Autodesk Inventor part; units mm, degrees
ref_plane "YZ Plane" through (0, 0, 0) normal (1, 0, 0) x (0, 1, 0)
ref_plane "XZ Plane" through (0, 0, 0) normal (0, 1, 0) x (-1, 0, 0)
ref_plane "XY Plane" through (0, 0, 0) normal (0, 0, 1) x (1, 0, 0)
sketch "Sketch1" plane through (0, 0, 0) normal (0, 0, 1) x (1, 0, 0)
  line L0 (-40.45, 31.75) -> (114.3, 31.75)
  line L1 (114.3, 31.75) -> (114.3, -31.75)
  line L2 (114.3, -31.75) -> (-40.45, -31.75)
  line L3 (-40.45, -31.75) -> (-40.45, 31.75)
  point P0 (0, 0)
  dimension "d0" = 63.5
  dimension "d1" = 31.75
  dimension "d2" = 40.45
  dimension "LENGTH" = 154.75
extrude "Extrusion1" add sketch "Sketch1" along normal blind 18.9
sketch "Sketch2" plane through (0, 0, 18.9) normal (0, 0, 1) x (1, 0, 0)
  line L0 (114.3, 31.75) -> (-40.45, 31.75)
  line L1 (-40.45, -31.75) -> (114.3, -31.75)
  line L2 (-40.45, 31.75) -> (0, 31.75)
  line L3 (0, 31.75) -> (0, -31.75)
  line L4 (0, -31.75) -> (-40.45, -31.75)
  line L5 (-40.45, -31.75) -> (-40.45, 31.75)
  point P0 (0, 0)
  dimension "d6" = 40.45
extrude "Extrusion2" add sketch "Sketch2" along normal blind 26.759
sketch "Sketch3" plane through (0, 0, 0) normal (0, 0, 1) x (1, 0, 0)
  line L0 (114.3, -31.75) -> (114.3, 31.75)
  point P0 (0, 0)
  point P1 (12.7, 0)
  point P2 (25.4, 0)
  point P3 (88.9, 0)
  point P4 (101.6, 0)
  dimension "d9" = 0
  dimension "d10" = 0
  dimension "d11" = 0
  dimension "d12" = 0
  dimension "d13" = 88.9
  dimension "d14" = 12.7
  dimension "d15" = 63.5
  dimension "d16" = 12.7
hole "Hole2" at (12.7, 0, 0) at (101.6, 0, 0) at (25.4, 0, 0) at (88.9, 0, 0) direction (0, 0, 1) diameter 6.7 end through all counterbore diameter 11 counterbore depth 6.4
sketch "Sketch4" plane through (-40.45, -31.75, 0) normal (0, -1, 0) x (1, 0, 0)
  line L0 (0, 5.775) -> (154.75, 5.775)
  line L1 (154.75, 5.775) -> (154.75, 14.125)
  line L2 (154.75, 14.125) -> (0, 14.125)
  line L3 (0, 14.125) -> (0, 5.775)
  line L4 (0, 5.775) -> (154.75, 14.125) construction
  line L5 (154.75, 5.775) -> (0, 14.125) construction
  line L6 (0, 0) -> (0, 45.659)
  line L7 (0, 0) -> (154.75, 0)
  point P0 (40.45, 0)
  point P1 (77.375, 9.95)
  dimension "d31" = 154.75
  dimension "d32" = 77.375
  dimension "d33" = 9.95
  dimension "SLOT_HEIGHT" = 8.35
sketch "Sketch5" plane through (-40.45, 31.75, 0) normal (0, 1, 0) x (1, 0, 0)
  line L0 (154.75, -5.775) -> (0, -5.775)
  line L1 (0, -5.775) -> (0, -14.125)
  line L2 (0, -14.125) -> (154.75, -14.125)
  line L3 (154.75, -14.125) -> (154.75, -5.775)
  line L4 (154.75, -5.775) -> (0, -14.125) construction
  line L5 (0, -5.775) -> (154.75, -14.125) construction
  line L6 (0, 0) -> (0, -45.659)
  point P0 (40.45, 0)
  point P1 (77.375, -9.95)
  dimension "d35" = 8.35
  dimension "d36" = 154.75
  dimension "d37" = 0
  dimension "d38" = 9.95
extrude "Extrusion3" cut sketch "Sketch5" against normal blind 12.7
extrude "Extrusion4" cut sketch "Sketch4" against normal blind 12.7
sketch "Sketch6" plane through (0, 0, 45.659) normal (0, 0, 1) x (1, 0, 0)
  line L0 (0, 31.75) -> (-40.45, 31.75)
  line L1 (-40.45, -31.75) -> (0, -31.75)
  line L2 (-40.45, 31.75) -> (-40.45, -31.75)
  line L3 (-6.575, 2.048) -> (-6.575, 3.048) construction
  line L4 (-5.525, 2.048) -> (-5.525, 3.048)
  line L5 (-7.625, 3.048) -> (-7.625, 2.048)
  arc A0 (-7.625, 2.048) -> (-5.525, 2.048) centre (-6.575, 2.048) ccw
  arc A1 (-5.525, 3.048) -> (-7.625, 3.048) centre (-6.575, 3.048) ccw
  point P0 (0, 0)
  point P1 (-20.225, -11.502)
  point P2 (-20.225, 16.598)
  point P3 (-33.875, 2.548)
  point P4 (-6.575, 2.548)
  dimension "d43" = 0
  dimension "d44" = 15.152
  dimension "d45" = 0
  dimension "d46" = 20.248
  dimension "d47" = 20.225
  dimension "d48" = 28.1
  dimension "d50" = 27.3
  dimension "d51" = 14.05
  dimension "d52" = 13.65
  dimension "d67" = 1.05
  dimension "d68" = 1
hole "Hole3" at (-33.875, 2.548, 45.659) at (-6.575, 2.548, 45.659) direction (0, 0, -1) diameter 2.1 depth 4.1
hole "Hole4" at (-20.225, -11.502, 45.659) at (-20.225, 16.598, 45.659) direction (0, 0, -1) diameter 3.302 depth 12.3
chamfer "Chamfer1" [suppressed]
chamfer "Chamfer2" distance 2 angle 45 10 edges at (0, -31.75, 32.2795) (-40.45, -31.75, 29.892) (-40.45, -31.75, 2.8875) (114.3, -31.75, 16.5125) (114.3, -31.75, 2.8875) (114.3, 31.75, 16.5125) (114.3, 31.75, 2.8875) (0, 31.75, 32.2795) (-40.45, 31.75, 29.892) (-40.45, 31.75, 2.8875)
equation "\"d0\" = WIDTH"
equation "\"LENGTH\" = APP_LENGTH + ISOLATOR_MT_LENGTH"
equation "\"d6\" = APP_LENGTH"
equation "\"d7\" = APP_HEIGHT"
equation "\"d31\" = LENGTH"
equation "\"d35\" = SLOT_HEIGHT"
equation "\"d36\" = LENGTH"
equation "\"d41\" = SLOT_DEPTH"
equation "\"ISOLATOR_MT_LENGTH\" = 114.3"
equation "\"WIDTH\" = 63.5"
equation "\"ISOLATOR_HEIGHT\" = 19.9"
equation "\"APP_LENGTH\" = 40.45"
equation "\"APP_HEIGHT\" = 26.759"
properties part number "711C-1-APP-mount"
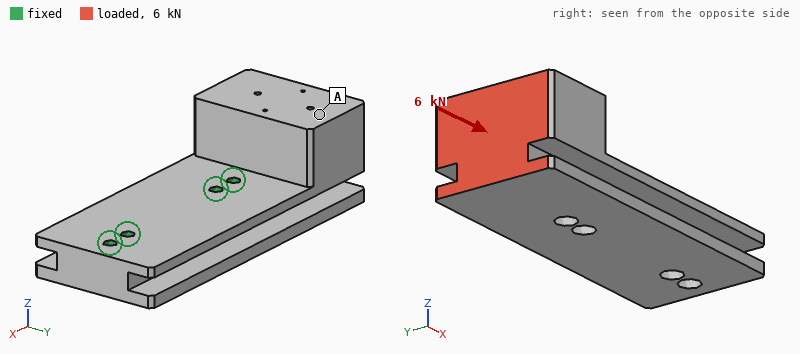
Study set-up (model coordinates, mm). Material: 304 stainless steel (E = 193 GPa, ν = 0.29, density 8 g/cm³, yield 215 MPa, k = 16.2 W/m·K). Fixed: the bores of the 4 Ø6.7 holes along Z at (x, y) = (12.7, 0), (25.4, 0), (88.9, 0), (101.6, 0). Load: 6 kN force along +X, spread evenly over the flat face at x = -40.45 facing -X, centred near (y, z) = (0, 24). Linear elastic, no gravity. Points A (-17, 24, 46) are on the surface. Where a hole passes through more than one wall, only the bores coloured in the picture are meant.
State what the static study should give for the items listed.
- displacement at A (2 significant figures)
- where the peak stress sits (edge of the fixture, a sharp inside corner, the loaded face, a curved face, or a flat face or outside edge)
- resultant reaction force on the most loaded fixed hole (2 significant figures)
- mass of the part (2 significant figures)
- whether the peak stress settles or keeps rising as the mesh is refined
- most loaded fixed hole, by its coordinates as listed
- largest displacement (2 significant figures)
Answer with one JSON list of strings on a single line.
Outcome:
["20 µm", "edge of the fixture", "4.9 kN", "1.7 kg", "keeps rising", "(12.7, 0)", "27 µm"]
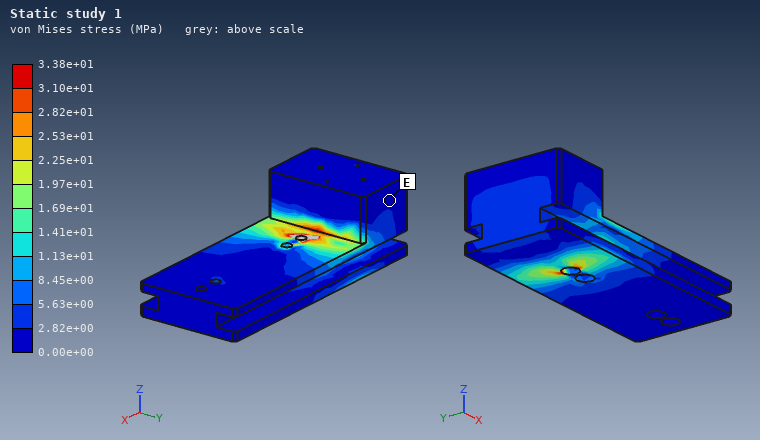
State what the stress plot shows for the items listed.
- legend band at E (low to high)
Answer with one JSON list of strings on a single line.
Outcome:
["0.00e+00 to 2.82e+00 MPa"]
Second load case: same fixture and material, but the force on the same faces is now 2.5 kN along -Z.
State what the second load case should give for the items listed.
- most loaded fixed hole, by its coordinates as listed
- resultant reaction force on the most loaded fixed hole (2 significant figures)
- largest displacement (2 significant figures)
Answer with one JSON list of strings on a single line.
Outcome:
["(12.7, 0)", "5.5 kN", "41 µm"]
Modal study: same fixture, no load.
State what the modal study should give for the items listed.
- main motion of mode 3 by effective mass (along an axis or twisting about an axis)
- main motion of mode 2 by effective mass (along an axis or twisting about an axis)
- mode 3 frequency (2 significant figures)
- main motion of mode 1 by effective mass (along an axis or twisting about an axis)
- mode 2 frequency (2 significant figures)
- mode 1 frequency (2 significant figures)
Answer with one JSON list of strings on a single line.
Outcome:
["along Y", "along Y", "4400 Hz", "along Z", "2600 Hz", "2000 Hz"]
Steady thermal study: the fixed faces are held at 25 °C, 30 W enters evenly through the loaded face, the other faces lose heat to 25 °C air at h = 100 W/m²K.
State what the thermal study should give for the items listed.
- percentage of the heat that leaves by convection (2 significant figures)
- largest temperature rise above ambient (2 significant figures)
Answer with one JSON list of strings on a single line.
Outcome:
["83 %", "32 K"]
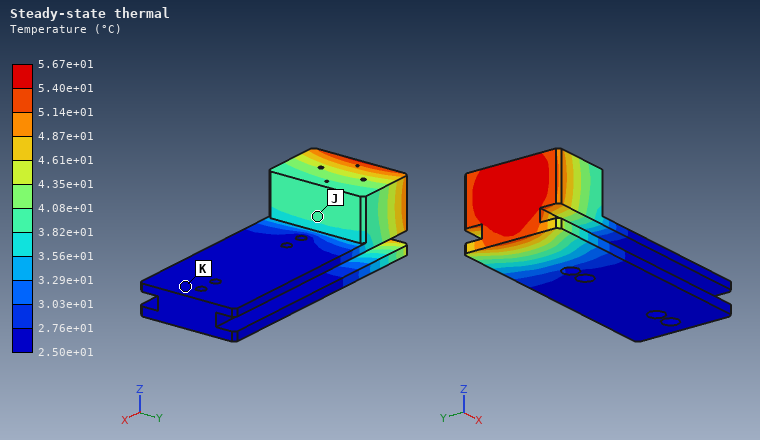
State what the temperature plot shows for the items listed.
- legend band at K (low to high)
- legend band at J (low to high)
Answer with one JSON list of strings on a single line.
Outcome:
["2.50e+01 to 2.76e+01 °C", "3.82e+01 to 4.08e+01 °C"]
